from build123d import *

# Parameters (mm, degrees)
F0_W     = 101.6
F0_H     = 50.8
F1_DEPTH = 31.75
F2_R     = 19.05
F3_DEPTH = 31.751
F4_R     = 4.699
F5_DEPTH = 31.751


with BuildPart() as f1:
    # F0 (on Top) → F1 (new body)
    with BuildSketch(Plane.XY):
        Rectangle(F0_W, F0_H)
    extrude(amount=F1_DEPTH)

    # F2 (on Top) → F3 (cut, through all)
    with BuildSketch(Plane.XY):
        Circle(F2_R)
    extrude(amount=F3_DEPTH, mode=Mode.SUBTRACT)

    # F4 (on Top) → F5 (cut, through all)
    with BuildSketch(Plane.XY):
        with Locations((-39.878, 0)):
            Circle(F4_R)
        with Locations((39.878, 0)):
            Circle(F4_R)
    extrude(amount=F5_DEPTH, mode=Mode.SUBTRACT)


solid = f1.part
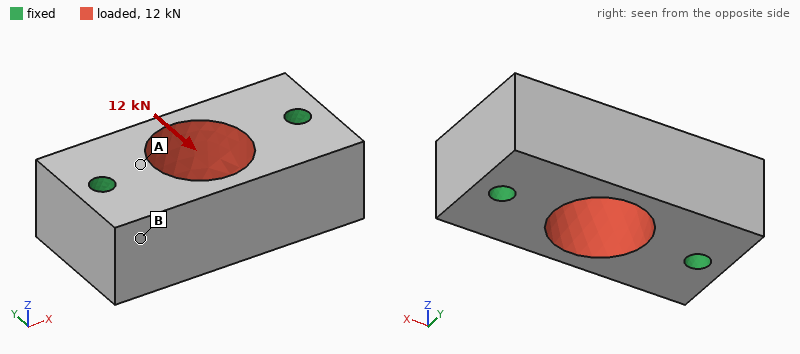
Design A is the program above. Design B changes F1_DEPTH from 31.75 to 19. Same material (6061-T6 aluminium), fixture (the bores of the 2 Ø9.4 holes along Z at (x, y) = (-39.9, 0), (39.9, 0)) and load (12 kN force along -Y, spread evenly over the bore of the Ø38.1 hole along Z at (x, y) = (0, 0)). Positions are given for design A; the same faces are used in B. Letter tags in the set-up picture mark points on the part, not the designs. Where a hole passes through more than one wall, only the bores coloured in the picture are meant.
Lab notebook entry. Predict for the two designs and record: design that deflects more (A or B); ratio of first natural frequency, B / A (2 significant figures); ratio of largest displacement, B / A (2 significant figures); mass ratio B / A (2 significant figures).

B
0.88
1.7
0.60
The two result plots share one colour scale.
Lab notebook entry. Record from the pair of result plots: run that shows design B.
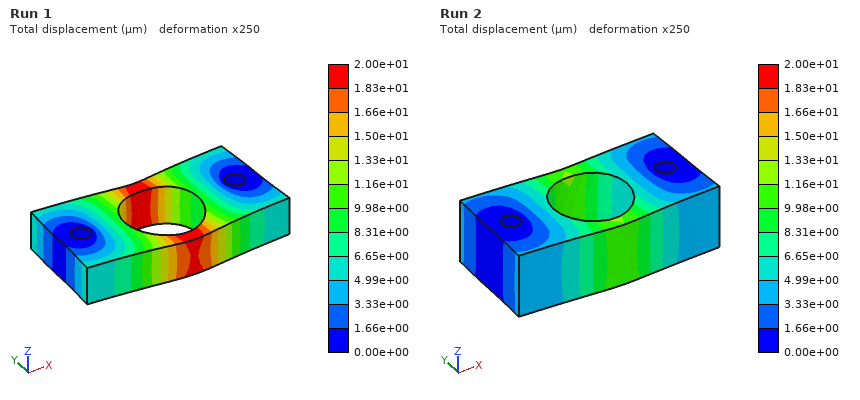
Run 1
